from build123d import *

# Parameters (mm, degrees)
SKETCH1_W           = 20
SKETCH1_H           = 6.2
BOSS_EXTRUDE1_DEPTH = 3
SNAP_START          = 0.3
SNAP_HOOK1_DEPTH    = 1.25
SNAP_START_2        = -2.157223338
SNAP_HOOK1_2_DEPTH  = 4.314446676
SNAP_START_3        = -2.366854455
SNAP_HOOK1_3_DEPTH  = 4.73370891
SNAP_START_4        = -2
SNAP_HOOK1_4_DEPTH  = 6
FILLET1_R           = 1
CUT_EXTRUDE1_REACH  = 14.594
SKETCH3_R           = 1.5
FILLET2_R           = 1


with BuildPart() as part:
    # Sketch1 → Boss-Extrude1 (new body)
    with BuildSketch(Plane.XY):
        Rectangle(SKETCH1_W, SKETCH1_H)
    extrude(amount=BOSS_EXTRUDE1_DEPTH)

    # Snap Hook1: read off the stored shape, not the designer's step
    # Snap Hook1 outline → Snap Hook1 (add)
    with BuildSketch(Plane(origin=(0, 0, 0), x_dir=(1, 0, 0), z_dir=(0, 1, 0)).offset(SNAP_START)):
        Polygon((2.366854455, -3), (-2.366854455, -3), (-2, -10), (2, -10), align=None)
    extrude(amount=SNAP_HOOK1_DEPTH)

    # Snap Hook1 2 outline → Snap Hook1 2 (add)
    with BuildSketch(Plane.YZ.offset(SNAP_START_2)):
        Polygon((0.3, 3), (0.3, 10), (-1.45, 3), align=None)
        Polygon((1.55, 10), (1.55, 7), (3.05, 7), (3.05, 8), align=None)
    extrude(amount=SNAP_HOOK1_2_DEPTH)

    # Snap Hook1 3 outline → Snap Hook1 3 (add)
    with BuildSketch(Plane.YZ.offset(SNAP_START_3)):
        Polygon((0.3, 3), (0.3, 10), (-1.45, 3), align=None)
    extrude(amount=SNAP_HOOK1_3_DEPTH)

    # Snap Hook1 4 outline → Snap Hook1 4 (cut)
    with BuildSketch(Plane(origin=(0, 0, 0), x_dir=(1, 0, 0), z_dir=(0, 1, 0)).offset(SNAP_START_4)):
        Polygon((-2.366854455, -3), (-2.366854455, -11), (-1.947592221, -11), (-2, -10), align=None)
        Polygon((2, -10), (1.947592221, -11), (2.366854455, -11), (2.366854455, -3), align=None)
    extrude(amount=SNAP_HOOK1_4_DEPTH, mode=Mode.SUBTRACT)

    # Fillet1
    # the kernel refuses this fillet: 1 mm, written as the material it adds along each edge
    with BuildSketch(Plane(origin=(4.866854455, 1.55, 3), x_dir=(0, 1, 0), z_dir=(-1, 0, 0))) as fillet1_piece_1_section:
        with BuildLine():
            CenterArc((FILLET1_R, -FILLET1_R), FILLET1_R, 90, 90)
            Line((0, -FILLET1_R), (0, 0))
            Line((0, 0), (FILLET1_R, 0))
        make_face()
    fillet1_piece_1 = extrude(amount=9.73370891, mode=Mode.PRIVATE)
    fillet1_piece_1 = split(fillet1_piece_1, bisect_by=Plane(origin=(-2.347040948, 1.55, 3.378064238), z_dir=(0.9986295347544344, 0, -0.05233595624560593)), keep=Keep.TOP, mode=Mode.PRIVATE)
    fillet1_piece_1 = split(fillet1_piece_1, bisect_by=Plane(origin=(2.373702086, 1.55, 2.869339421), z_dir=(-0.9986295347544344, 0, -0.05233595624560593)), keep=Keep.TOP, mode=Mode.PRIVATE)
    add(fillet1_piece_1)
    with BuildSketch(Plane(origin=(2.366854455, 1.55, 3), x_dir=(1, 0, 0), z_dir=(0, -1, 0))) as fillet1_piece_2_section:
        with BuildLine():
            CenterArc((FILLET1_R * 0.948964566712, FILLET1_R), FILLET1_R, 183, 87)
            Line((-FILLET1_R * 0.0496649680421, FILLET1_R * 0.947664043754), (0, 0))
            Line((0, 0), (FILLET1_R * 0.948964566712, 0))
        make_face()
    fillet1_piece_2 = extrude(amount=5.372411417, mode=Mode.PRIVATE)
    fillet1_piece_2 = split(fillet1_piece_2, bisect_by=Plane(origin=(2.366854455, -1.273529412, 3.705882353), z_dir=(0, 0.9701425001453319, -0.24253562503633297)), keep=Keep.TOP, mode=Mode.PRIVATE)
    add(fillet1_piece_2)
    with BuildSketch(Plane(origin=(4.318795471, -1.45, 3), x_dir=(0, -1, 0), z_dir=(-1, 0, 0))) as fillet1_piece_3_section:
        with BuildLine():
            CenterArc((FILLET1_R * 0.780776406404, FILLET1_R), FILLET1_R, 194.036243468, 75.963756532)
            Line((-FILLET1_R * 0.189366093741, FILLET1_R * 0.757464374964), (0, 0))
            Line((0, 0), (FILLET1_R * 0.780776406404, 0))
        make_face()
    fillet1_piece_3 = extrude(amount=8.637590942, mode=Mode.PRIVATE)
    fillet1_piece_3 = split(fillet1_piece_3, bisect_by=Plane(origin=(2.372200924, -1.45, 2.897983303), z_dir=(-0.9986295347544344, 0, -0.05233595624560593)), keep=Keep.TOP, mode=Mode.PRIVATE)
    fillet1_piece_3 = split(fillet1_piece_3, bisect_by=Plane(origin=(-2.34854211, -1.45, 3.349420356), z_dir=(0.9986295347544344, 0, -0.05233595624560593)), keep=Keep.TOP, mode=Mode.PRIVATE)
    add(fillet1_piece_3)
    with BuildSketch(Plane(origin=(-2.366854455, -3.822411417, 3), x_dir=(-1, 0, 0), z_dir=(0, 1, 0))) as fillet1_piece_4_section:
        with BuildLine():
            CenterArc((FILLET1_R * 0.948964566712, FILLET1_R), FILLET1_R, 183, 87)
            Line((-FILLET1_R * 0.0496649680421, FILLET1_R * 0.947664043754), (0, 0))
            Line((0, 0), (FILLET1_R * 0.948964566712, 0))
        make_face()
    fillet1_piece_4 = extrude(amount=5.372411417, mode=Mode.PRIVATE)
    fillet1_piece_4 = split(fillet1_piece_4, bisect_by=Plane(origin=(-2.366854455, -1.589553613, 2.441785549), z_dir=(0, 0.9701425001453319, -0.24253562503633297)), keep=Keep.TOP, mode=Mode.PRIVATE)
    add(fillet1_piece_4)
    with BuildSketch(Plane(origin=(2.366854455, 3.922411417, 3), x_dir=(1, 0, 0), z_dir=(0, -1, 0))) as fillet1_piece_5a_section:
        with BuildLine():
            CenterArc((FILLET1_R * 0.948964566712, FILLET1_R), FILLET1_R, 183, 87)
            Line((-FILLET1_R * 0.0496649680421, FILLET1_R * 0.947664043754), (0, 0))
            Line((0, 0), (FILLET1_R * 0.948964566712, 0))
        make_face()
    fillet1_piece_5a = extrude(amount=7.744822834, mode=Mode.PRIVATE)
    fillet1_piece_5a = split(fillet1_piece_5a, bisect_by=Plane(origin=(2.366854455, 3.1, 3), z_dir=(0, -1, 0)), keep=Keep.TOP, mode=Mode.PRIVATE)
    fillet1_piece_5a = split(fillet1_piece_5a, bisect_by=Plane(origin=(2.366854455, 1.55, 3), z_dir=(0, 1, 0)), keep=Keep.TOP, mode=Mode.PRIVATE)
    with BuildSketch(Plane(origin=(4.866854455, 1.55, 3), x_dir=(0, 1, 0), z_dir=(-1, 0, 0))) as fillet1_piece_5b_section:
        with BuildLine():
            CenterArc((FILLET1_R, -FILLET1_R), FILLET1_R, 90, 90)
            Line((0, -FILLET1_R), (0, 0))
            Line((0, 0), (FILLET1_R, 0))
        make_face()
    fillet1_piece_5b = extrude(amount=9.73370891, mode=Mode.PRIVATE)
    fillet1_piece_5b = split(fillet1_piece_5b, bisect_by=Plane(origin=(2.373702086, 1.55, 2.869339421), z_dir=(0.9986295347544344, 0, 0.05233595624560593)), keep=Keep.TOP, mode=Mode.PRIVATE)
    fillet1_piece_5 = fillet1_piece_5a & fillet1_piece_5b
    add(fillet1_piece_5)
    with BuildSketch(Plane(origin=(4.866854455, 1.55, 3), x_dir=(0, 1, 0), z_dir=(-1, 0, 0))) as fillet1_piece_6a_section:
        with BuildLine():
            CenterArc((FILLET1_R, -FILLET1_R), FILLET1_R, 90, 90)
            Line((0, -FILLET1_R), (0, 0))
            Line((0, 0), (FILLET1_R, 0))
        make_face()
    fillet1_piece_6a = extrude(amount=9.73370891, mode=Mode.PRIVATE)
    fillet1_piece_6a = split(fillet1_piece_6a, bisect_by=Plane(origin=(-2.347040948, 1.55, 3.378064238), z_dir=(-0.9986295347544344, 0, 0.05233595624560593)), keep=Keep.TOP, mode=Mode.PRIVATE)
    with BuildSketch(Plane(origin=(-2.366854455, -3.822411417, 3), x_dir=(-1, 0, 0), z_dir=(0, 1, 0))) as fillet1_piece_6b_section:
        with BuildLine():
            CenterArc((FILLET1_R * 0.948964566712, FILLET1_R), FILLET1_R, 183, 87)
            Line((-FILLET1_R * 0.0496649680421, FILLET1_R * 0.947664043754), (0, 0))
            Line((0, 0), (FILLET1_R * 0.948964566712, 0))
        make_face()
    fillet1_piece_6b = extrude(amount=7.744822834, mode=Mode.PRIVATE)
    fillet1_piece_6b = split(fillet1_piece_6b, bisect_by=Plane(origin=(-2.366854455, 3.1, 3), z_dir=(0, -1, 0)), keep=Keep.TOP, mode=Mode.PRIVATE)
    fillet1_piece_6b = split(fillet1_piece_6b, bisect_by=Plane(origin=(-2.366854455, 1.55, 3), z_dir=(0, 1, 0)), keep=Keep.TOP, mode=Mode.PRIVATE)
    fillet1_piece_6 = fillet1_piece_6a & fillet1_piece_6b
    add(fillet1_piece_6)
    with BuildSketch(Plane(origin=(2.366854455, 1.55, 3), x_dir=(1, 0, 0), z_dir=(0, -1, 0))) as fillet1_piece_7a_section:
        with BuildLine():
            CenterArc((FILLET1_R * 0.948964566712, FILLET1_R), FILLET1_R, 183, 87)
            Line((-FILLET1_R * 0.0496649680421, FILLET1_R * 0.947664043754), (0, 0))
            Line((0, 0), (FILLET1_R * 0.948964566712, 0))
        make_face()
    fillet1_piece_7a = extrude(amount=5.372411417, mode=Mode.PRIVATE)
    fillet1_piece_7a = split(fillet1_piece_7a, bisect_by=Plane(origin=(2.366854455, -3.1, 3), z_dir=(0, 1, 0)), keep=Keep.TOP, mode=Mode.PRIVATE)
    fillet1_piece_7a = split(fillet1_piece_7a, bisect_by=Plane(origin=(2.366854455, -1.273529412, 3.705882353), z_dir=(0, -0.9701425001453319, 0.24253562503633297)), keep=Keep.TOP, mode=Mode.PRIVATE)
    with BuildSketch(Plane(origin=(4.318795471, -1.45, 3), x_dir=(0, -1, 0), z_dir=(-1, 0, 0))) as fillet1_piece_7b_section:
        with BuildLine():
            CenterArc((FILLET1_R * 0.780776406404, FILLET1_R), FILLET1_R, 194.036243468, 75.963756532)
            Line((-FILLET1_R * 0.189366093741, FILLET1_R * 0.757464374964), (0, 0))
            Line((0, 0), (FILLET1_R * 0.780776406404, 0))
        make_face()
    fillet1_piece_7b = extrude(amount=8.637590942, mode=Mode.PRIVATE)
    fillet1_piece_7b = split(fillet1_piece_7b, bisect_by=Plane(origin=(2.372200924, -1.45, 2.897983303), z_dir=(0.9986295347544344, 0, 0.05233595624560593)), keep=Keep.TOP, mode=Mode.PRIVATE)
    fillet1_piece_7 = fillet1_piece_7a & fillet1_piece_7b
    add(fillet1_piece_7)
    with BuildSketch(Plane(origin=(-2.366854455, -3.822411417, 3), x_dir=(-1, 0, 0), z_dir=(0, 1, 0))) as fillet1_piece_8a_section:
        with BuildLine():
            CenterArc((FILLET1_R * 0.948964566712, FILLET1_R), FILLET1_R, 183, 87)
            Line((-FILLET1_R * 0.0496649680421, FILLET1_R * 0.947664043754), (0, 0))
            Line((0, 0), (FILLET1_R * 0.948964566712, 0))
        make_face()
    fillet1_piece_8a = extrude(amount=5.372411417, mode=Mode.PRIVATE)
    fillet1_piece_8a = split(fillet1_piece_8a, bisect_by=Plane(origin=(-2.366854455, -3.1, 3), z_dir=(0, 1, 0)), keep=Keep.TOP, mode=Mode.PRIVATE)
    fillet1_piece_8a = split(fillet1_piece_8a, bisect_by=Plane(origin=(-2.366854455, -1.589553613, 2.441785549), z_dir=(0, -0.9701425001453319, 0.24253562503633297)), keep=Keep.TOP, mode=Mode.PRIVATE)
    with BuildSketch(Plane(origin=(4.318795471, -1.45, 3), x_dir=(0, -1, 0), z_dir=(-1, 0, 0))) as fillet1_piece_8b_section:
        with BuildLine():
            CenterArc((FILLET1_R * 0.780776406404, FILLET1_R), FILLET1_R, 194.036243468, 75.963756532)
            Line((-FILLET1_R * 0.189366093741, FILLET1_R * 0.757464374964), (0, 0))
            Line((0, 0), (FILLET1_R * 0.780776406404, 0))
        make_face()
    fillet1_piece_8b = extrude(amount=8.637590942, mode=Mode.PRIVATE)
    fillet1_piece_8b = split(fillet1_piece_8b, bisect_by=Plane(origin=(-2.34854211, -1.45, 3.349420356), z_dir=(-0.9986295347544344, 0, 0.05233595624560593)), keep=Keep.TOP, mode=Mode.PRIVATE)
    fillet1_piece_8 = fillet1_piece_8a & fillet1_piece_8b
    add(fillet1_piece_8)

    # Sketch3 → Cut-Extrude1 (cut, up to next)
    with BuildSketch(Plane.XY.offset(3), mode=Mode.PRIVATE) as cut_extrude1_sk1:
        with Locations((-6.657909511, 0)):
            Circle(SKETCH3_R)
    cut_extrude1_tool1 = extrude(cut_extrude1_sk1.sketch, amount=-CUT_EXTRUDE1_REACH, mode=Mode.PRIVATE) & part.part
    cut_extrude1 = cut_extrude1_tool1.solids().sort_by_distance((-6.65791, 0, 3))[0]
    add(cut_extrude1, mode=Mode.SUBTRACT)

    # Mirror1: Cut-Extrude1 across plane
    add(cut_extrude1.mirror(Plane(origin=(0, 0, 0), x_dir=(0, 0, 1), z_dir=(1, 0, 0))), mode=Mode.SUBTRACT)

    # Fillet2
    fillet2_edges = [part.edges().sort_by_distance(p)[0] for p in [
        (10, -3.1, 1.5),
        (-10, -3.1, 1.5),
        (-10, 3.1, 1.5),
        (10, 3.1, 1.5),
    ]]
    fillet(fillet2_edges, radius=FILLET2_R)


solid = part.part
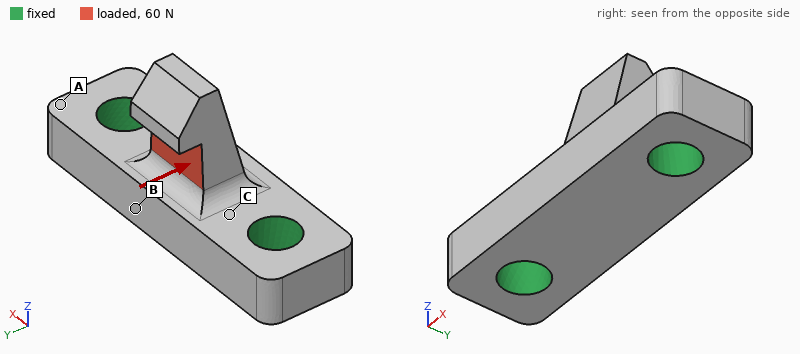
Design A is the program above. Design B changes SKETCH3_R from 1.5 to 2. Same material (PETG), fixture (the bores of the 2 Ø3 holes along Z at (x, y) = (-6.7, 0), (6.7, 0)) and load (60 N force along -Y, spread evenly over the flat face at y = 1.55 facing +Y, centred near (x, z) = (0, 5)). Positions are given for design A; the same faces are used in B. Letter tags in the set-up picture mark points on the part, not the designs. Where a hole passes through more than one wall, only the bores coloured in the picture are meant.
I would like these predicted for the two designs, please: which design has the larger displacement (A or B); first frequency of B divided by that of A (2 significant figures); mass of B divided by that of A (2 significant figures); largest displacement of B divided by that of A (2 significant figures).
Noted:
A
1.1
0.92
0.89
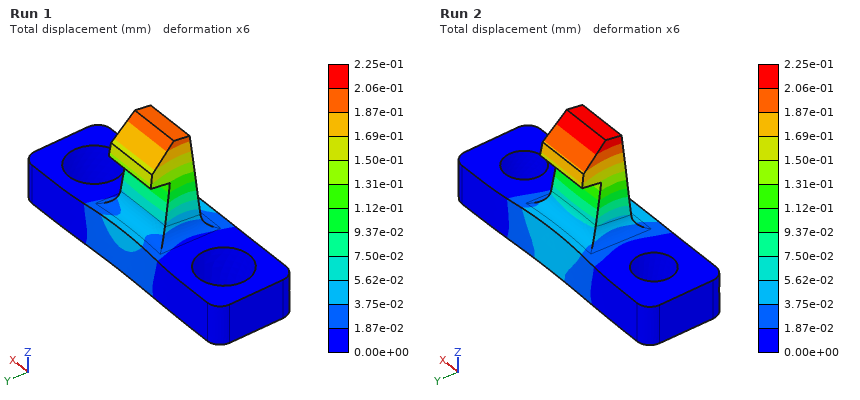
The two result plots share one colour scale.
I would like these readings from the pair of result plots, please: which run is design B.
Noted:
Run 1
